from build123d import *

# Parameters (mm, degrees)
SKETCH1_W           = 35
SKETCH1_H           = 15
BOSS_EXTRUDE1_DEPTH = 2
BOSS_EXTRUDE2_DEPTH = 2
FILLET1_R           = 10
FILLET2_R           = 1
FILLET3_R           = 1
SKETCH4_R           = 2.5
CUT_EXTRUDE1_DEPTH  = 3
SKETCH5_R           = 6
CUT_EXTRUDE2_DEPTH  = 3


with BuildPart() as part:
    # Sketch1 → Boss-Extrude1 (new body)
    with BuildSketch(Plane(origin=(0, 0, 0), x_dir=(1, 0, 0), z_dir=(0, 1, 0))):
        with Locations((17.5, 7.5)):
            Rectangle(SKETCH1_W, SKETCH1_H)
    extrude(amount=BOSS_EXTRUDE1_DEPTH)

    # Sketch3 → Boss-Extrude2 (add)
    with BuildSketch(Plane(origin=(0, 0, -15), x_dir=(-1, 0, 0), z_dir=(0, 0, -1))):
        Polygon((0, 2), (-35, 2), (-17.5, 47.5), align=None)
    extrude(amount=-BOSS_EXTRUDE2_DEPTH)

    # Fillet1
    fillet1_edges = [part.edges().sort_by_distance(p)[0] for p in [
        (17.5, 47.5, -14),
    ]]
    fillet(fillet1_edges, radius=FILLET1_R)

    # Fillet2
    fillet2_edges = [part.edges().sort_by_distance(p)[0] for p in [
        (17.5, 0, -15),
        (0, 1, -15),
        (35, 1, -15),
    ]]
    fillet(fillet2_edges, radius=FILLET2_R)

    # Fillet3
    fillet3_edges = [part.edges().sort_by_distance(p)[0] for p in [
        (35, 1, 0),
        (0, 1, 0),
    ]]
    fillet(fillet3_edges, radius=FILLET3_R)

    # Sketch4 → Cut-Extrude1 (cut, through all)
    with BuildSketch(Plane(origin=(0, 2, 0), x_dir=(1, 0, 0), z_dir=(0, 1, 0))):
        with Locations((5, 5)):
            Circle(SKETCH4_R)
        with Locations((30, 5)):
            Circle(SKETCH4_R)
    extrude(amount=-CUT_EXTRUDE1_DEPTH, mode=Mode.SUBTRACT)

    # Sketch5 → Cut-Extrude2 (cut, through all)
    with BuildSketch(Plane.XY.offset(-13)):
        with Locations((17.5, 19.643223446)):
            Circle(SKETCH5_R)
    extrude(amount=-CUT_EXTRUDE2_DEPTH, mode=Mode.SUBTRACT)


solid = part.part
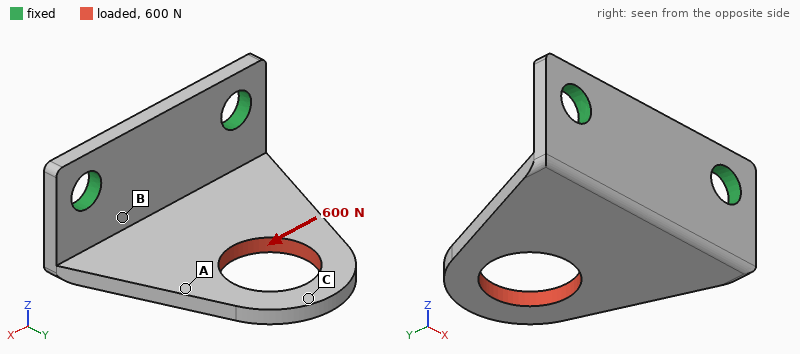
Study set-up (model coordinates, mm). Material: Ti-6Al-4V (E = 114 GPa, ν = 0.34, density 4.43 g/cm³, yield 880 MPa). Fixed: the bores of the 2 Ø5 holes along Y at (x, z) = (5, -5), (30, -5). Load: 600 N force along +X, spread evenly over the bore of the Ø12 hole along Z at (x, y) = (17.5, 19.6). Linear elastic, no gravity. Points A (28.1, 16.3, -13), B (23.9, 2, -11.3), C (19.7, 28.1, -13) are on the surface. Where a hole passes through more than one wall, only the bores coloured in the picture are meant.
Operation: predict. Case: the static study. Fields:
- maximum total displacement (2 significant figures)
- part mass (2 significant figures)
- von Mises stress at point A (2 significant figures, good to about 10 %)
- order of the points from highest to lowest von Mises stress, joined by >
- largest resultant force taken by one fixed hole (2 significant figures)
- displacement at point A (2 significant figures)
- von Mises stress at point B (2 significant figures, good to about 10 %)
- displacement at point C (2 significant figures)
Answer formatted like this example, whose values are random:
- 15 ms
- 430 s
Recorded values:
- 0.11 mm
- 9.1 g
- 55 MPa
- B > A > C
- 550 N
- 0.080 mm
- 98 MPa
- 0.11 mm
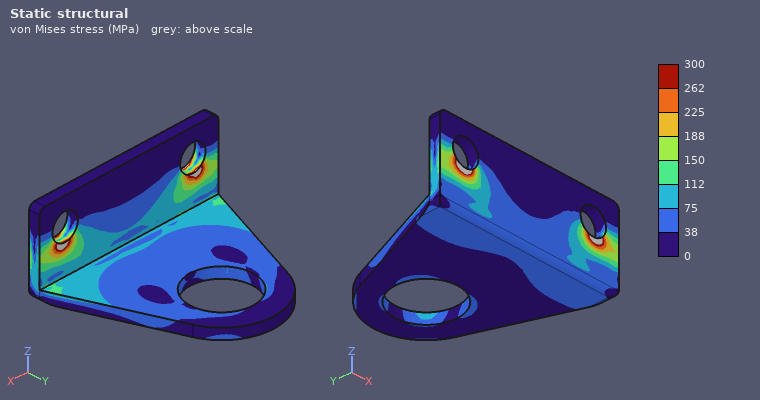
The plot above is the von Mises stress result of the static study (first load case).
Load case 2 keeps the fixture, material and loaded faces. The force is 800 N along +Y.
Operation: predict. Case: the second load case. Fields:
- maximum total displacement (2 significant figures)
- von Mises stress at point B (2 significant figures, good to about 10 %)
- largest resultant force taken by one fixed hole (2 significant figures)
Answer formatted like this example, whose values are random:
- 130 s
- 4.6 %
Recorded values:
- 0.26 mm
- 79 MPa
- 400 N
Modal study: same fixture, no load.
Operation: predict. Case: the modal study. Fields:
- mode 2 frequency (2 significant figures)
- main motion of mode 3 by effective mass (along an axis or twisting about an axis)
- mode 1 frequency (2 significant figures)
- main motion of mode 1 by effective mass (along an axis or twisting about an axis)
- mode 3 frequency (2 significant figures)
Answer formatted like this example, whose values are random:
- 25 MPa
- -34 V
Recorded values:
- 6300 Hz
- along Y
- 2300 Hz
- along Z
- 8200 Hz
